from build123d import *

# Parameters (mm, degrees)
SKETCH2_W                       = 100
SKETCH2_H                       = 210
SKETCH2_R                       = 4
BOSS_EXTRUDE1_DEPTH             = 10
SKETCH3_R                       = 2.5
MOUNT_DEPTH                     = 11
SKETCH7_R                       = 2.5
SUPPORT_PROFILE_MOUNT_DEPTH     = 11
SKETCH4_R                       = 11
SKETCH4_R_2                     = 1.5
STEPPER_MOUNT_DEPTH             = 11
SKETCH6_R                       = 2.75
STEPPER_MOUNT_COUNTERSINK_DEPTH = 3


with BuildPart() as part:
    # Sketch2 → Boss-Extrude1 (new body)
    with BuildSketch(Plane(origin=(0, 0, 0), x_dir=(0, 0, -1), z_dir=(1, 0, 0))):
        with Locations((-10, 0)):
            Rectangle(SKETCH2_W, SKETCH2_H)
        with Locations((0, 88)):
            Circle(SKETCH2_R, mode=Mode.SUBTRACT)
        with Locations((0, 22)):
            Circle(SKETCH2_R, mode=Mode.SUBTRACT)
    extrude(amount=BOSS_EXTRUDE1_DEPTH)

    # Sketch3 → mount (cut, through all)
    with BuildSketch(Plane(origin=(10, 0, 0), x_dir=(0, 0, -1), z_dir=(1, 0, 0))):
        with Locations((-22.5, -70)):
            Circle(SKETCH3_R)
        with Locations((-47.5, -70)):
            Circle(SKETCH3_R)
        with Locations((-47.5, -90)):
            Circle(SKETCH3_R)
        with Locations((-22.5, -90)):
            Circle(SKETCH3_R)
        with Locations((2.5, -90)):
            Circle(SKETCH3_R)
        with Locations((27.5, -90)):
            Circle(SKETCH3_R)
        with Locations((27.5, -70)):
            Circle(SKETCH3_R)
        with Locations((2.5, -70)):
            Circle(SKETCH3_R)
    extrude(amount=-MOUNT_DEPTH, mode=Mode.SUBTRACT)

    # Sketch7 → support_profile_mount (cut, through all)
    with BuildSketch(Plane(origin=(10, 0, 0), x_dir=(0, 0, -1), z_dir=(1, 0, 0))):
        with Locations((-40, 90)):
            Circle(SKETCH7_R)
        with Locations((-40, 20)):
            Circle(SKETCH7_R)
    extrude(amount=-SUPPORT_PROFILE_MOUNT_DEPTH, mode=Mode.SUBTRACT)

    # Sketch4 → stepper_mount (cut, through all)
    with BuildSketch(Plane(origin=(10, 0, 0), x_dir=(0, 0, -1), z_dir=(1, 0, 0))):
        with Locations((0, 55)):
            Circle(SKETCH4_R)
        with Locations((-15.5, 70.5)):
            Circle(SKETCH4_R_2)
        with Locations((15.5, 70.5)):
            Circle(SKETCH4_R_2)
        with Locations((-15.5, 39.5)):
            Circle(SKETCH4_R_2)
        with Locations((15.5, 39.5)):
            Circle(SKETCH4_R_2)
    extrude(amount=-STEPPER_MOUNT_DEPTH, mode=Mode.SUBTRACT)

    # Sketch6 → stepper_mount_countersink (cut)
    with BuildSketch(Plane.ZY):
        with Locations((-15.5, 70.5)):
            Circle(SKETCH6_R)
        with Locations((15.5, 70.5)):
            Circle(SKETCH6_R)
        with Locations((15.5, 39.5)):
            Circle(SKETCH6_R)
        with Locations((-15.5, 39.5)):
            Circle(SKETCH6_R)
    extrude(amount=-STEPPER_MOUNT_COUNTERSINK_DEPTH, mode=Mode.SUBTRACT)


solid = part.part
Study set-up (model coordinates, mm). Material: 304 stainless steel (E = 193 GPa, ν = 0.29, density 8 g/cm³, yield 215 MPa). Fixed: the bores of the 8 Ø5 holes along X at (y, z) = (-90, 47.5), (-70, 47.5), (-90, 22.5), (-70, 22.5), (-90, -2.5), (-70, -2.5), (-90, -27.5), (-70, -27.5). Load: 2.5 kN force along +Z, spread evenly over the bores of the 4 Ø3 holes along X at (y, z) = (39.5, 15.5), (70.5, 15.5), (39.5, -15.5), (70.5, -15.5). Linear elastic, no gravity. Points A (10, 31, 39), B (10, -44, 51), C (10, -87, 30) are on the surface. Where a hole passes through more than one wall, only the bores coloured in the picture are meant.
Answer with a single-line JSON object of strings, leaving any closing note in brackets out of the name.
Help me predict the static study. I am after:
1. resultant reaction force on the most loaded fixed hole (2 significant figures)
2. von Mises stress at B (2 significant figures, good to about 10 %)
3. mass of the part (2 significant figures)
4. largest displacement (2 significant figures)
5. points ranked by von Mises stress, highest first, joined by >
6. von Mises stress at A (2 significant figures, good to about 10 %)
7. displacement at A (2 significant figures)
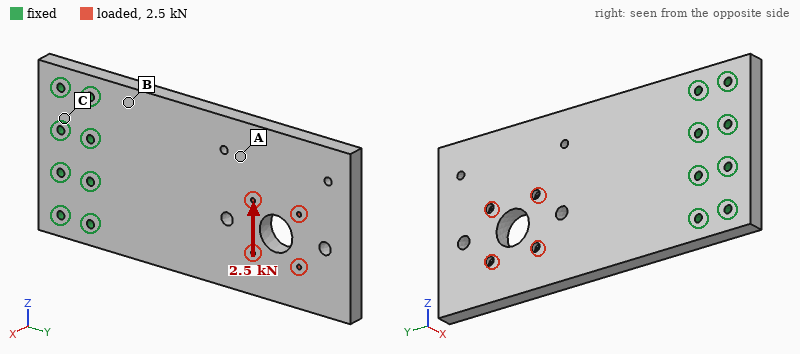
{"resultant reaction force on the most loaded fixed hole": "3.0 kN", "von Mises stress at B": "12 MPa", "mass of the part": "1.6 kg", "largest displacement": "27 µm", "points ranked by von Mises stress, highest first, joined by >": "B > A > C", "von Mises stress at A": "5.9 MPa", "displacement at A": "14 µm"}
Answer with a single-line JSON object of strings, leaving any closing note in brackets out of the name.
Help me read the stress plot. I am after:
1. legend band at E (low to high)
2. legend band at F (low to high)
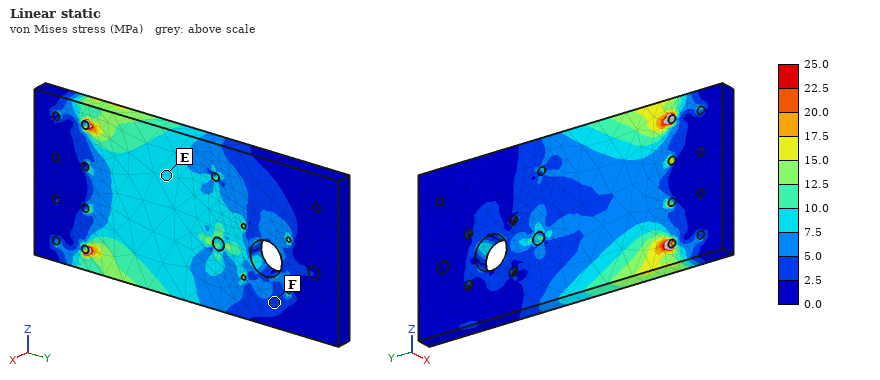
{"legend band at E": "7.5 to 10.0 MPa", "legend band at F": "2.5 to 5.0 MPa"}
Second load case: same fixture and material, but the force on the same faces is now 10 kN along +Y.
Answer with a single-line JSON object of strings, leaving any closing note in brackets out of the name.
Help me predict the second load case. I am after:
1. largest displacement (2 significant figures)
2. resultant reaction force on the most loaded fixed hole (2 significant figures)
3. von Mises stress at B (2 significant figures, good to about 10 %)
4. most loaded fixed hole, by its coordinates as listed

{"largest displacement": "0.13 mm", "resultant reaction force on the most loaded fixed hole": "3.1 kN", "von Mises stress at B": "14 MPa", "most loaded fixed hole, by its coordinates as listed": "(-70, -27.5)"}
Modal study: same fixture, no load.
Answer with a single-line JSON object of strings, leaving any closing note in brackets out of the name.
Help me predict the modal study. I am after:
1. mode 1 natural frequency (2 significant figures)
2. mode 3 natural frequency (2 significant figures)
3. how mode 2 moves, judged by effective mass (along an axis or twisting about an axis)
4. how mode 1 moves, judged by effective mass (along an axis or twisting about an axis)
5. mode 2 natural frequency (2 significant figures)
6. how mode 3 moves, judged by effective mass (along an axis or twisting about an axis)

{"mode 1 natural frequency": "270 Hz", "mode 3 natural frequency": "1600 Hz", "how mode 2 moves, judged by effective mass": "twisting about Y", "how mode 1 moves, judged by effective mass": "along X", "mode 2 natural frequency": "960 Hz", "how mode 3 moves, judged by effective mass": "along X"}
